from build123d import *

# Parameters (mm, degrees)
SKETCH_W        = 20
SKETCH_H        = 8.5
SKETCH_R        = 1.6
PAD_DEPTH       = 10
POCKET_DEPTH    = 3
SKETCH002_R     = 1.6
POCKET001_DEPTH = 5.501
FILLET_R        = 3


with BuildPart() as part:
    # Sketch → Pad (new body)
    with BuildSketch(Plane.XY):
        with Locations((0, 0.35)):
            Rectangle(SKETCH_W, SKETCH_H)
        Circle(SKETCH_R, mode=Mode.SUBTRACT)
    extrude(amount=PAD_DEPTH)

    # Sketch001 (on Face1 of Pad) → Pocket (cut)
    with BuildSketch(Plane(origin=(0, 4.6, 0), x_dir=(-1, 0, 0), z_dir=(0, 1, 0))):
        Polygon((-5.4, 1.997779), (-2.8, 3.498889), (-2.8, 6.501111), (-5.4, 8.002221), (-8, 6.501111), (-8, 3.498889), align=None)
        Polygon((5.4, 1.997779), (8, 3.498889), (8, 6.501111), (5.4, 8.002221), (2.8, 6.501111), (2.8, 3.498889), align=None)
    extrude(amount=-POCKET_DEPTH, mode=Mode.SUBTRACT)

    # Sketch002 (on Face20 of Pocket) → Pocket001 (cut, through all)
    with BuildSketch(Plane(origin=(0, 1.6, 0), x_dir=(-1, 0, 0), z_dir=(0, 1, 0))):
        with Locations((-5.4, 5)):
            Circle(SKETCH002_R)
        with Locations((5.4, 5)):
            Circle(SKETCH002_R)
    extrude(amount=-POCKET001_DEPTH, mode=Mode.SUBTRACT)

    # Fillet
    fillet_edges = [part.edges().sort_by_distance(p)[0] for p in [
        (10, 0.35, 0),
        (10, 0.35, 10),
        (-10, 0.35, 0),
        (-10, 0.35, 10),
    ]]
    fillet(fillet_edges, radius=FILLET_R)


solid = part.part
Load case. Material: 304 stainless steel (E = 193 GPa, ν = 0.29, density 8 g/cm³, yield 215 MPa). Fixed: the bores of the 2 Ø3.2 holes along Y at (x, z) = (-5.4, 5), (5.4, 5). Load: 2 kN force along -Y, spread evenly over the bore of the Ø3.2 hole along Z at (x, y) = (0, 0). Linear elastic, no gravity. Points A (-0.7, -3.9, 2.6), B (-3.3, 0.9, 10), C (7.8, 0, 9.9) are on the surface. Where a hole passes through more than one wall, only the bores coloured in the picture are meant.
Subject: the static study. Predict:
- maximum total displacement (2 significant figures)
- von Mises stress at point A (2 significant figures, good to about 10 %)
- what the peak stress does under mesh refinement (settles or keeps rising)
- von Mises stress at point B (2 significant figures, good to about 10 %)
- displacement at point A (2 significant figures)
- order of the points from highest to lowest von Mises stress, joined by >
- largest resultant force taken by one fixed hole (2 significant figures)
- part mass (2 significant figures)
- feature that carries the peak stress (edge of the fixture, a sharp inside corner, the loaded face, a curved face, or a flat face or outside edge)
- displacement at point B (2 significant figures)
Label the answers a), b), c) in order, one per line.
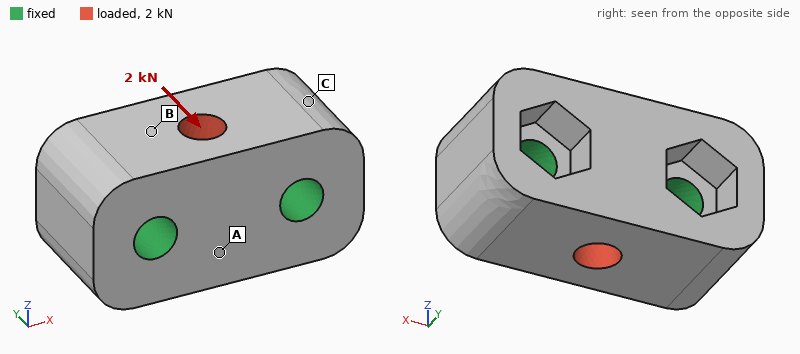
a) 1.5 µm
b) 27 MPa
c) keeps rising
d) 17 MPa
e) 1.0 µm
f) A > B > C
g) 1.0 kN
h) 11 g
i) edge of the fixture
j) 0.78 µm
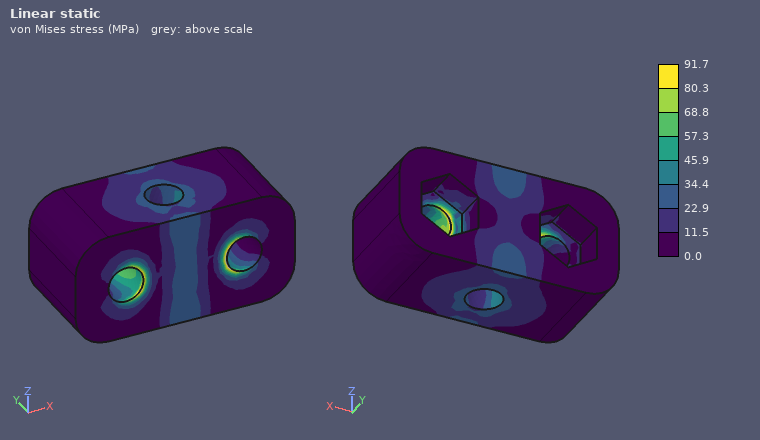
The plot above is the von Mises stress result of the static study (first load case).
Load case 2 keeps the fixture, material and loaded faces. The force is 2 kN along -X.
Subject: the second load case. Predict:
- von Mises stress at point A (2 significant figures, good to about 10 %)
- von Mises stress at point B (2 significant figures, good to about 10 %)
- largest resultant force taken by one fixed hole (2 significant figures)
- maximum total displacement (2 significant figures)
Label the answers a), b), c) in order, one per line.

a) 7.7 MPa
b) 16 MPa
c) 1.0 kN
d) 0.73 µm
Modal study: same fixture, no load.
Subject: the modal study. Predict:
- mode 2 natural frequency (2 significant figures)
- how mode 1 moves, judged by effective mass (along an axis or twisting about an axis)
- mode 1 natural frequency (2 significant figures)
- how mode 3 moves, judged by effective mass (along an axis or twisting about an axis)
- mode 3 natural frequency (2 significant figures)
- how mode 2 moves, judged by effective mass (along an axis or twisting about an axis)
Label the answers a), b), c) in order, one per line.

a) 87 kHz
b) along Z
c) 69 kHz
d) along X
e) 93 kHz
f) twisting about Y
